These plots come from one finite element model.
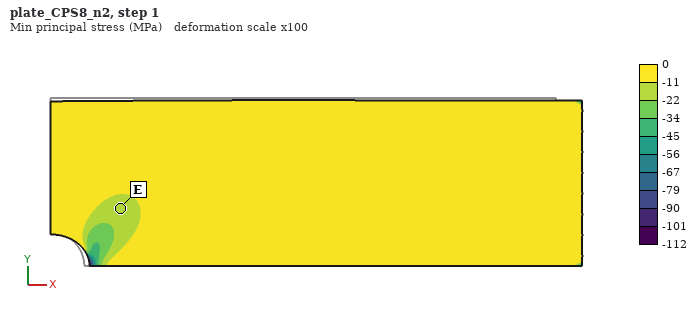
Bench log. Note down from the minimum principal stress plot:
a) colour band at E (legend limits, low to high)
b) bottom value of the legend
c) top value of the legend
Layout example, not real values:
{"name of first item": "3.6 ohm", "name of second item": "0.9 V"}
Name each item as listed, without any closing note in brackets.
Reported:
{"colour band at E": "-22 to -11 MPa", "bottom value of the legend": "-112 MPa", "top value of the legend": "0 MPa"}
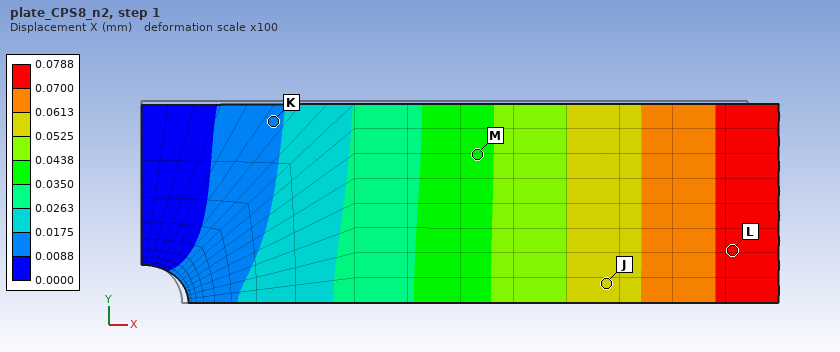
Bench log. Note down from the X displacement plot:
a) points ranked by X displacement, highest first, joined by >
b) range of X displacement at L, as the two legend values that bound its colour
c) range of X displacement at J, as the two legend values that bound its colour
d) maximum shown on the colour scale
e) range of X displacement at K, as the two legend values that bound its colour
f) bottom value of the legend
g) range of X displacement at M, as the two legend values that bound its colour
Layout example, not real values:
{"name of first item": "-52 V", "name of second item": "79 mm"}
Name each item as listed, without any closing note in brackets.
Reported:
{"points ranked by X displacement, highest first, joined by >": "L > J > M > K", "range of X displacement at L, as the two legend values that bound its colour": "0.0700 to 0.0788 mm", "range of X displacement at J, as the two legend values that bound its colour": "0.0525 to 0.0613 mm", "maximum shown on the colour scale": "0.0788 mm", "range of X displacement at K, as the two legend values that bound its colour": "0.0088 to 0.0175 mm", "bottom value of the legend": "0.0000 mm", "range of X displacement at M, as the two legend values that bound its colour": "0.0350 to 0.0438 mm"}
